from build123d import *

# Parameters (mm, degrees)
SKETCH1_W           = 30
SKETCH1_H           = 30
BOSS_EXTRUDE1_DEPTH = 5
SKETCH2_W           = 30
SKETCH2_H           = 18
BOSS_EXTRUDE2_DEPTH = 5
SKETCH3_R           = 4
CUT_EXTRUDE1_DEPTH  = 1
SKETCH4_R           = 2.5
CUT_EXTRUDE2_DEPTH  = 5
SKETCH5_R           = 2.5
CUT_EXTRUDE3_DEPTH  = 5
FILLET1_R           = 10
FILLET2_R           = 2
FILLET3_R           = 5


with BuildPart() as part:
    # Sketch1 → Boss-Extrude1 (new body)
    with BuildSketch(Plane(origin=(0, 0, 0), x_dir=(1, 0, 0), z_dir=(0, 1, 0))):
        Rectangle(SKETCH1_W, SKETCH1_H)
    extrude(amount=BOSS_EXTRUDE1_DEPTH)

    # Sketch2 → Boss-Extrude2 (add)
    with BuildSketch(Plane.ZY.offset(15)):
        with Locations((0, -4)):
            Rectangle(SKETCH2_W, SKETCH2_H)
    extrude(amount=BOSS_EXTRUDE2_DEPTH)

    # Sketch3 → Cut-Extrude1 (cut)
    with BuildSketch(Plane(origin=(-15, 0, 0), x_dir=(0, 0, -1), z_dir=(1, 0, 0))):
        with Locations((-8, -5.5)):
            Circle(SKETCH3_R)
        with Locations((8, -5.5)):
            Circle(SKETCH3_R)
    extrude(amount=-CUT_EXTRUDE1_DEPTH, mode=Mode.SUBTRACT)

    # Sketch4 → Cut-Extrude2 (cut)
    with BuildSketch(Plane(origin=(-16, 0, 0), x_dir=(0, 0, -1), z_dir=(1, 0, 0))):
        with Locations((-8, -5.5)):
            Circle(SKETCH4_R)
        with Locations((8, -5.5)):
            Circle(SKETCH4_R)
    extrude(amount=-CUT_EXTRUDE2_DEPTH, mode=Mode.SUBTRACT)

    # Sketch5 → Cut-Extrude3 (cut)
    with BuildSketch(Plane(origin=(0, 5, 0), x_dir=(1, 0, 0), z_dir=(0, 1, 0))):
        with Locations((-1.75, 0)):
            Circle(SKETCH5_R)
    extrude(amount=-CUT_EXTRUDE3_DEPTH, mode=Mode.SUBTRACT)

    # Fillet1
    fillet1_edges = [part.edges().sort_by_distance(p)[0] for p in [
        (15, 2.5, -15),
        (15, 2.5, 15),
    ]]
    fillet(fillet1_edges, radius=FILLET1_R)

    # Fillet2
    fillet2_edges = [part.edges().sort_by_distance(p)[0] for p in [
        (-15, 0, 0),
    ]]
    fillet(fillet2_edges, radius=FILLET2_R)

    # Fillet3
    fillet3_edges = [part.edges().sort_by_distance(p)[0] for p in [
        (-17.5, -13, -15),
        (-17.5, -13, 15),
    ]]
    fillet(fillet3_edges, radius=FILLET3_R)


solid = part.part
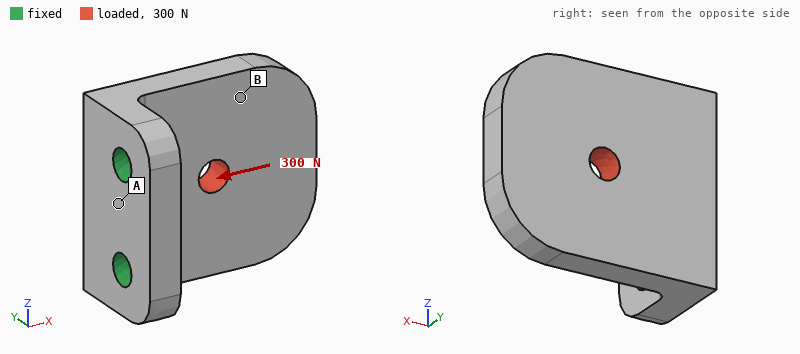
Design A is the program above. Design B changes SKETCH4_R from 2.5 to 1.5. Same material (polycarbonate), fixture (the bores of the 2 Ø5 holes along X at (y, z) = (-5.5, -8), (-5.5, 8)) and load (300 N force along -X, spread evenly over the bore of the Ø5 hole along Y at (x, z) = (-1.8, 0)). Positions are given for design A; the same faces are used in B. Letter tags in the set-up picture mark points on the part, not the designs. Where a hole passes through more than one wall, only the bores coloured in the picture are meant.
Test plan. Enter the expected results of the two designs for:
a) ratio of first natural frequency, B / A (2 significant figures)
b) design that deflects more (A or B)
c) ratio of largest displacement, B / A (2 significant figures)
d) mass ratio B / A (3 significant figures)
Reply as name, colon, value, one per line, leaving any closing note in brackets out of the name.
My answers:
ratio of first natural frequency, B / A: 0.90
design that deflects more: B
ratio of largest displacement, B / A: 1.5
mass ratio B / A: 1.02
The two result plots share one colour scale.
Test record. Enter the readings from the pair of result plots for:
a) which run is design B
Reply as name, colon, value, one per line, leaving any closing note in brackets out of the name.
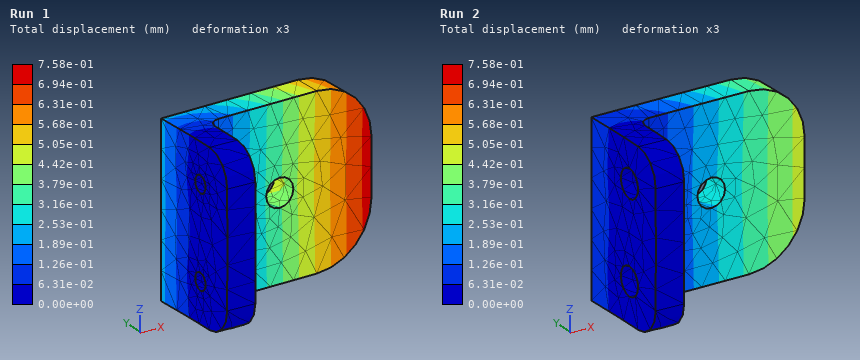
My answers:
which run is design B: Run 1
